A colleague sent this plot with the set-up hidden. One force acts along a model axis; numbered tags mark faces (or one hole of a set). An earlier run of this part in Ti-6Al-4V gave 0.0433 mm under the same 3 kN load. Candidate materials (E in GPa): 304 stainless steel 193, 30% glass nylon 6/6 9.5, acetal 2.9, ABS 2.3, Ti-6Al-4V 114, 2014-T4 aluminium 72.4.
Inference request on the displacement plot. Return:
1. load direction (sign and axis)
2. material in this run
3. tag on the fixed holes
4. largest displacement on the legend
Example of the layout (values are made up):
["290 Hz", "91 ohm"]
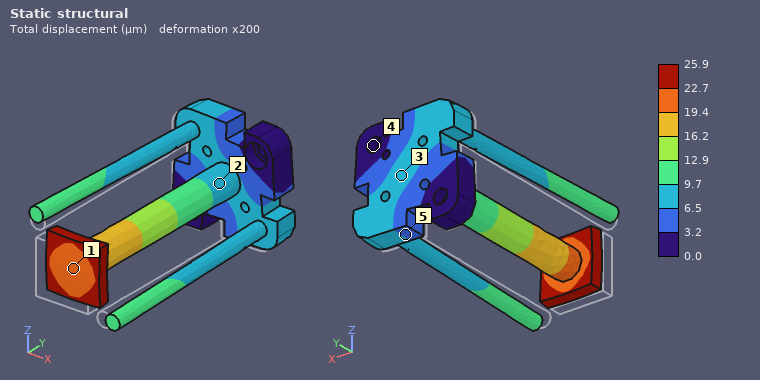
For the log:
["+Y", "304 stainless steel", "4", "25.9 µm"]
